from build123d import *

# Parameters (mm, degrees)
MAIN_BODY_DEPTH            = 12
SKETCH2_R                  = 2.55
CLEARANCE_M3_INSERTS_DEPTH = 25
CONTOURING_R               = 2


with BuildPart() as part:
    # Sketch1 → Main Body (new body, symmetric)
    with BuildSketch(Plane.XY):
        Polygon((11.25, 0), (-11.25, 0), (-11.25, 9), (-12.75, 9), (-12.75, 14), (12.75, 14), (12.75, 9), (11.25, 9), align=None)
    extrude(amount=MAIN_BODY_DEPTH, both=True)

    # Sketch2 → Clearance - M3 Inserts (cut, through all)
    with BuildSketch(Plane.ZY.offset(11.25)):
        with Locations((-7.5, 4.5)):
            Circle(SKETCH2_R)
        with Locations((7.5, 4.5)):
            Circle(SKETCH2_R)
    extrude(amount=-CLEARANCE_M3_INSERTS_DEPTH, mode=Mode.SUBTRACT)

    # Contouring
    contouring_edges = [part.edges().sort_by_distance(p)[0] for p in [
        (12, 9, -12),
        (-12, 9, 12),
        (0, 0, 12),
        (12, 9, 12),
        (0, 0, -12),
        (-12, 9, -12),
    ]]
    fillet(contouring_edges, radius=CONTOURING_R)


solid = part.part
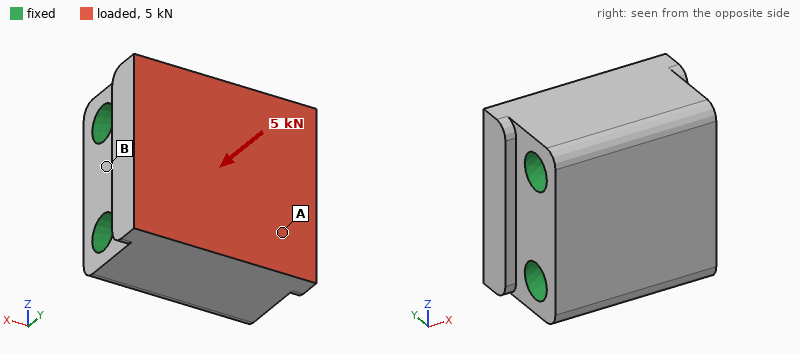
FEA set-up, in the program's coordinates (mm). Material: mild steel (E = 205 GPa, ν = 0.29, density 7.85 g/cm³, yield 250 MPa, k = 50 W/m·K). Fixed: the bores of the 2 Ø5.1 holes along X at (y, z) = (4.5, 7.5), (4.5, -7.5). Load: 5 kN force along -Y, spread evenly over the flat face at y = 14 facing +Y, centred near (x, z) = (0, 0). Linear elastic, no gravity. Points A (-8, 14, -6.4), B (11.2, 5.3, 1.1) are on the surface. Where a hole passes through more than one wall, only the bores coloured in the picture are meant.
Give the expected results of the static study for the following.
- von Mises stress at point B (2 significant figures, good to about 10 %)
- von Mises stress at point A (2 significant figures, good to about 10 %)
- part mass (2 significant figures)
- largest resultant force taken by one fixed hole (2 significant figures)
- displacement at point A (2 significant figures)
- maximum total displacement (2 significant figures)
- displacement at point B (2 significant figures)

4.9 MPa
11 MPa
55 g
2.5 kN
0.42 µm
0.70 µm
0.26 µm
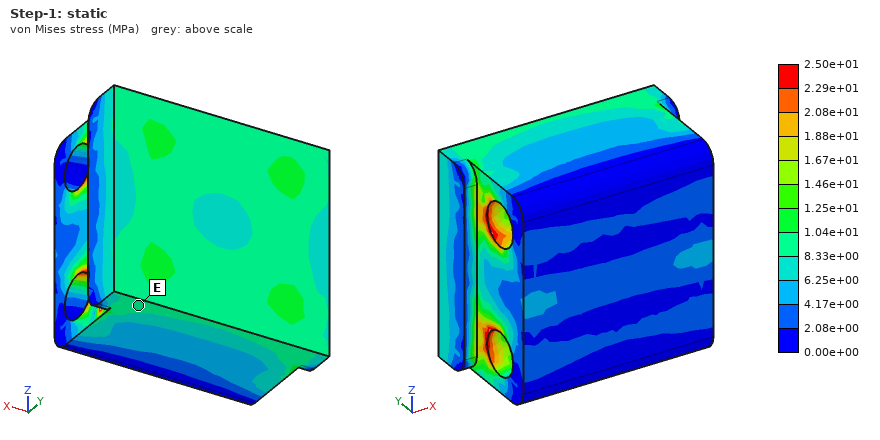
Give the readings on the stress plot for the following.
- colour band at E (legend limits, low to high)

8.33e+00 to 1.04e+01 MPa
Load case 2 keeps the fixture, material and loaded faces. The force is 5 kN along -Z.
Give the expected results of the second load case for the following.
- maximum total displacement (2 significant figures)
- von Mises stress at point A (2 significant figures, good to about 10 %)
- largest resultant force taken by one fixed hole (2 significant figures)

1.9 µm
18 MPa
3.3 kN
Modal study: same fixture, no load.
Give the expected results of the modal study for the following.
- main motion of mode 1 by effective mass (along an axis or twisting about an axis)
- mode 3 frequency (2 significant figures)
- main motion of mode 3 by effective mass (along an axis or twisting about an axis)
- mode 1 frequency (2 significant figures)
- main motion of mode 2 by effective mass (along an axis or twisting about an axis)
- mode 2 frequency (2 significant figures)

along X
84 kHz
twisting about Y
73 kHz
along Z
79 kHz
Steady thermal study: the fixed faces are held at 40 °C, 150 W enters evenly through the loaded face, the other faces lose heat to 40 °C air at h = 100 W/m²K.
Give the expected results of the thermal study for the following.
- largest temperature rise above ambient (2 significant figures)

47 K
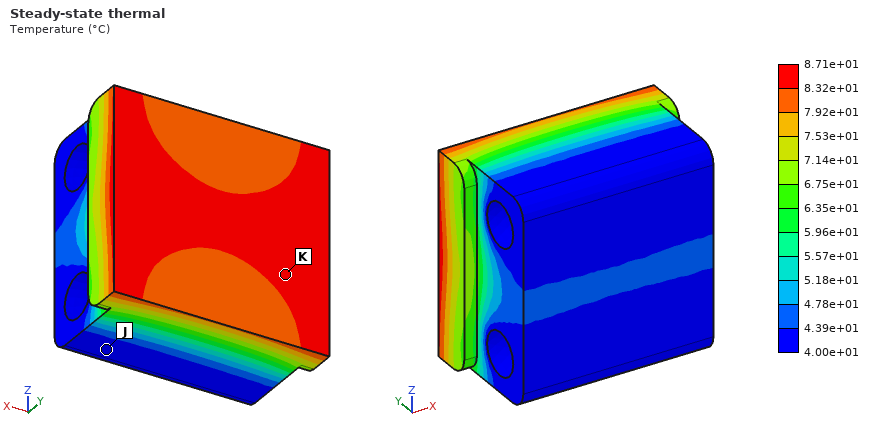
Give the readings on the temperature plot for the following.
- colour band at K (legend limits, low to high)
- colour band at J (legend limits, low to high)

8.32e+01 to 8.71e+01 °C
4.00e+01 to 4.39e+01 °C
